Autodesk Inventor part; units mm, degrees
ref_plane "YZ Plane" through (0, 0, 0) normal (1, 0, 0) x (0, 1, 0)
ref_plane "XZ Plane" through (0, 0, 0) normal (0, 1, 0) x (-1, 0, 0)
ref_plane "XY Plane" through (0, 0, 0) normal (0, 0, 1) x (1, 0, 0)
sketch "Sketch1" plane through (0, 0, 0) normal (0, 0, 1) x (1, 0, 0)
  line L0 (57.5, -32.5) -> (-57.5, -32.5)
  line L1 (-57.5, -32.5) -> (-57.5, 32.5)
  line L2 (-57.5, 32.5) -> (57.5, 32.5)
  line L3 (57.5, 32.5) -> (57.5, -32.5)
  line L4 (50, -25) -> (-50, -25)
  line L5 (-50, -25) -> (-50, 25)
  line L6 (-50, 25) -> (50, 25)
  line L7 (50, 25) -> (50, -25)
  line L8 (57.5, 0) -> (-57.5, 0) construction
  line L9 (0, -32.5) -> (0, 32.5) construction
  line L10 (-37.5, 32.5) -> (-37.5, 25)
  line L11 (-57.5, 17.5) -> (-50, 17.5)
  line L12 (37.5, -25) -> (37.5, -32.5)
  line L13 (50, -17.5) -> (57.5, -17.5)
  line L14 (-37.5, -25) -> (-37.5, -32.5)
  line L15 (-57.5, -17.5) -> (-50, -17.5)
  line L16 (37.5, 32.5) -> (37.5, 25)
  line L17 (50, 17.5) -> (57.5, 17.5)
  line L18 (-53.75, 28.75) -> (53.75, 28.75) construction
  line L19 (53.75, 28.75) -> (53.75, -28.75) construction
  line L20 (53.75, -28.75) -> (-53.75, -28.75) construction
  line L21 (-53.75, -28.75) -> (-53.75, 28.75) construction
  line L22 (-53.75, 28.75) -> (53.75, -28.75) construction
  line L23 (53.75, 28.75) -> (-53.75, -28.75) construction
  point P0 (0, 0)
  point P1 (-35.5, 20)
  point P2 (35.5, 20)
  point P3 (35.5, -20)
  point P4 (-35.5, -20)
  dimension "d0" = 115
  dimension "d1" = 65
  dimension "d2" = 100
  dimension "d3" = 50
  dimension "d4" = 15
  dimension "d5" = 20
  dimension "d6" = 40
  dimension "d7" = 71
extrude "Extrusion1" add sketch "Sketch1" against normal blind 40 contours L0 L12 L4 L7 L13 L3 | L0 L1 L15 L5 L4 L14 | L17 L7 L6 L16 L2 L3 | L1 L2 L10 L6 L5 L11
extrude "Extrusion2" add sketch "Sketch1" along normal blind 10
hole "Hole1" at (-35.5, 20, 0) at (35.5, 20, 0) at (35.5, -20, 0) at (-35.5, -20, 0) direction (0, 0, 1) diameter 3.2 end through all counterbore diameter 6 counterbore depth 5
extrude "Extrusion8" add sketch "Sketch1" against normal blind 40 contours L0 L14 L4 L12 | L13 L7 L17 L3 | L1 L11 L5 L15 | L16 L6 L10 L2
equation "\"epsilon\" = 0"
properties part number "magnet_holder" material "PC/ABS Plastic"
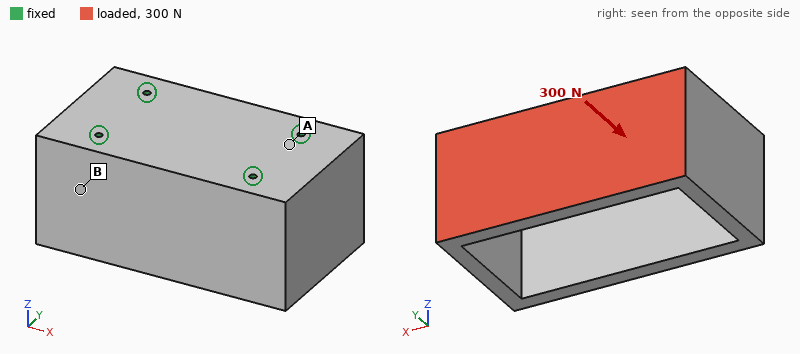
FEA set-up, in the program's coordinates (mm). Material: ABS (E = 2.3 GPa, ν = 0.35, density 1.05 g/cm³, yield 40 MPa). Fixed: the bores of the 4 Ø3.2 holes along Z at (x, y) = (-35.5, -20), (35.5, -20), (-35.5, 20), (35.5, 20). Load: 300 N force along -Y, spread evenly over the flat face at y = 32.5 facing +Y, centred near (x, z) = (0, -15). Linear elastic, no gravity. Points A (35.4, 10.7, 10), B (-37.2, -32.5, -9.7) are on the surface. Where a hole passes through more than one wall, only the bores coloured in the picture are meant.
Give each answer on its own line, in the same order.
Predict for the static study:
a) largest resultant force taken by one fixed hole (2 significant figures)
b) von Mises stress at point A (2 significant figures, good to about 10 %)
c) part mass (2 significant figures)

110 N
0.59 MPa
180 g
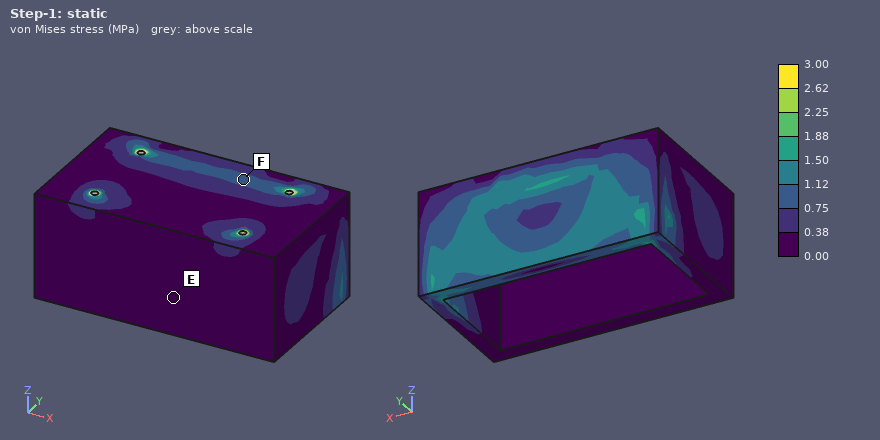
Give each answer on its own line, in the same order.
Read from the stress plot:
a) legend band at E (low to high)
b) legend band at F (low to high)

0.00 to 0.38 MPa
0.75 to 1.12 MPa
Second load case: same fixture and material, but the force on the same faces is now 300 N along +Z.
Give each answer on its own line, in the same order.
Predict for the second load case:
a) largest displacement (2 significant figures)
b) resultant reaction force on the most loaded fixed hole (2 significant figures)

100 µm
190 N
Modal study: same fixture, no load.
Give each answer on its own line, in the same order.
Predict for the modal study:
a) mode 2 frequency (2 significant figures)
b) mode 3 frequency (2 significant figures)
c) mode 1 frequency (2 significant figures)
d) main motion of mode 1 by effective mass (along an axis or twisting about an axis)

1200 Hz
1300 Hz
1100 Hz
along Y
